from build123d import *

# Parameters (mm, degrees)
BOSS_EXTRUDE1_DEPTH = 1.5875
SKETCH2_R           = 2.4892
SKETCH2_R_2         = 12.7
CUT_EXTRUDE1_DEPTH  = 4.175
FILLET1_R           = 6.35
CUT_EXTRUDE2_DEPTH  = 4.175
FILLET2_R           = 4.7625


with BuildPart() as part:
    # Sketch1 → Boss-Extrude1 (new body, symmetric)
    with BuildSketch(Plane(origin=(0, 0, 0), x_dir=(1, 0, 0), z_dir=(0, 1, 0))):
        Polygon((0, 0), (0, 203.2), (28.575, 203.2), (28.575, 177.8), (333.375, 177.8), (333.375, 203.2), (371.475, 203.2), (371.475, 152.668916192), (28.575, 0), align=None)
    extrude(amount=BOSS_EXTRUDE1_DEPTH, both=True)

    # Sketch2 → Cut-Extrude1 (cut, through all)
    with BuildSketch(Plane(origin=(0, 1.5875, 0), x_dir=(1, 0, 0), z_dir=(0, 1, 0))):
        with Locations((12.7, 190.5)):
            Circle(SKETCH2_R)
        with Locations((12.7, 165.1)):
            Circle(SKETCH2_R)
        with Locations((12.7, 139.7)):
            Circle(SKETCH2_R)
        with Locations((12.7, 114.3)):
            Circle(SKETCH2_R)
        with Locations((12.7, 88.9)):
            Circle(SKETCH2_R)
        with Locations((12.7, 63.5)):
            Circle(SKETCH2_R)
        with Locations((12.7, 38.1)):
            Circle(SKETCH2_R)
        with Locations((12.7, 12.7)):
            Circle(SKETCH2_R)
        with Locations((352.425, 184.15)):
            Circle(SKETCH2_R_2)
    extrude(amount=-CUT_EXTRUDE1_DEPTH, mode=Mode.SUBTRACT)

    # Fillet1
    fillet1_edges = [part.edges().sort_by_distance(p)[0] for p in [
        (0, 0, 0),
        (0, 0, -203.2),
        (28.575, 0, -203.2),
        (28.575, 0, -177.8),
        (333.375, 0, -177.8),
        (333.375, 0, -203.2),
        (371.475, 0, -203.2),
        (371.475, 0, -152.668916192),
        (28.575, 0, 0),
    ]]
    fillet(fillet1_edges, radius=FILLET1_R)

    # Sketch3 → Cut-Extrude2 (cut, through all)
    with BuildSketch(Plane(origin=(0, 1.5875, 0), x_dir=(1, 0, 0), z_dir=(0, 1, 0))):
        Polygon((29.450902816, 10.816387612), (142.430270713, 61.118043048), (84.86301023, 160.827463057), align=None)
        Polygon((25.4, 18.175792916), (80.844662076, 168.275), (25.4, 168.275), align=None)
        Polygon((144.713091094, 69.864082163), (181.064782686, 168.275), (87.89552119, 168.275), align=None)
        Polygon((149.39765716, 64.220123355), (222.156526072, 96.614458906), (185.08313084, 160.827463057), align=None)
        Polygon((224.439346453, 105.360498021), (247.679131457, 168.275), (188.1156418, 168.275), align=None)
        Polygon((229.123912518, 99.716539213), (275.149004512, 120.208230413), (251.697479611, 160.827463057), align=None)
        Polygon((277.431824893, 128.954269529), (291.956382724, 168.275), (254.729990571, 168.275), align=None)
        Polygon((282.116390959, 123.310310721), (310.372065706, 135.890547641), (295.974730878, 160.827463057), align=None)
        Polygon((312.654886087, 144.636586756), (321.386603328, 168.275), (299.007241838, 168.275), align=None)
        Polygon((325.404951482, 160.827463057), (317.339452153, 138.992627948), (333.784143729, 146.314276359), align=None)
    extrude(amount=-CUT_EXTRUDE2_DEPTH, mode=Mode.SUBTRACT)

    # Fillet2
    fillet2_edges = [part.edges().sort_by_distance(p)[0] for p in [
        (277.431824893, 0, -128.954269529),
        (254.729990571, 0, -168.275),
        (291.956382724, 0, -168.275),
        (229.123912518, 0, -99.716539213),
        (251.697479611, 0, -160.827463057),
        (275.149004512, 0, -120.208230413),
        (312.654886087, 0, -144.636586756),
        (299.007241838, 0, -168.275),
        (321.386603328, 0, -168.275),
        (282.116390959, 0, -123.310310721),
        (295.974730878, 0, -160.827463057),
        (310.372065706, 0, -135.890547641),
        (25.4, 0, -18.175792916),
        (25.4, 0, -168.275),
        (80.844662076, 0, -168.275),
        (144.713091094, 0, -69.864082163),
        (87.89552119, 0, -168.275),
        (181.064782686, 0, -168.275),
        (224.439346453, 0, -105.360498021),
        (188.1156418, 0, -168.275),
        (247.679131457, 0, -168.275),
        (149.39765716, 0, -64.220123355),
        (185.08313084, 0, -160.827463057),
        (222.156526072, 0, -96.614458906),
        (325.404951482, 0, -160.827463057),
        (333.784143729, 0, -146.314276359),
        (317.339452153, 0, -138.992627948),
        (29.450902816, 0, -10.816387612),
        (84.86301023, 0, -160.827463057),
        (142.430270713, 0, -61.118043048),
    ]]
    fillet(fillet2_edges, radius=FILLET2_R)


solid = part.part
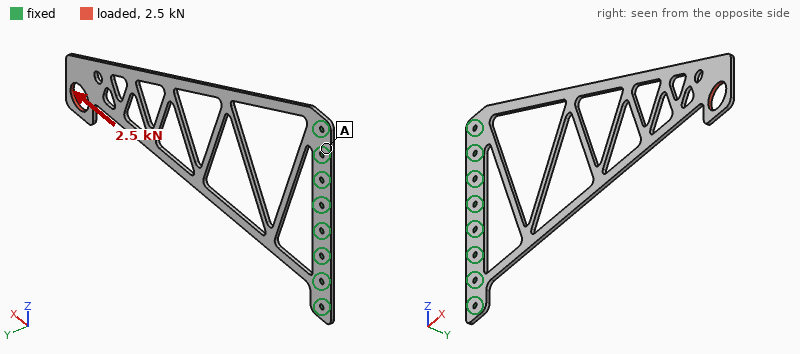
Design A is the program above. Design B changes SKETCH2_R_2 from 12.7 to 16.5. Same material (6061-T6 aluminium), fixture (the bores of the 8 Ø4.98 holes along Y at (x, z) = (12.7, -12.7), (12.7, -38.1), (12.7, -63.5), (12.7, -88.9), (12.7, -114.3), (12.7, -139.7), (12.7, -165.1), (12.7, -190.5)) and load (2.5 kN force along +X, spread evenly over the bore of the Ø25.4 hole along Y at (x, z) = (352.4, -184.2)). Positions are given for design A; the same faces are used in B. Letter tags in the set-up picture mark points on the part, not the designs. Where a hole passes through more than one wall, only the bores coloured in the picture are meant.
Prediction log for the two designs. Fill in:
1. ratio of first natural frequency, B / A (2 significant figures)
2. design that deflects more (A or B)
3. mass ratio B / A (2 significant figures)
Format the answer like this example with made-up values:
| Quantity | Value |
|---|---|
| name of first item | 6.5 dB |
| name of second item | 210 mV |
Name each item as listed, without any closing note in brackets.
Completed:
| Quantity | Value |
|---|---|
| ratio of first natural frequency, B / A | 1.0 |
| design that deflects more | B |
| mass ratio B / A | 0.98 |
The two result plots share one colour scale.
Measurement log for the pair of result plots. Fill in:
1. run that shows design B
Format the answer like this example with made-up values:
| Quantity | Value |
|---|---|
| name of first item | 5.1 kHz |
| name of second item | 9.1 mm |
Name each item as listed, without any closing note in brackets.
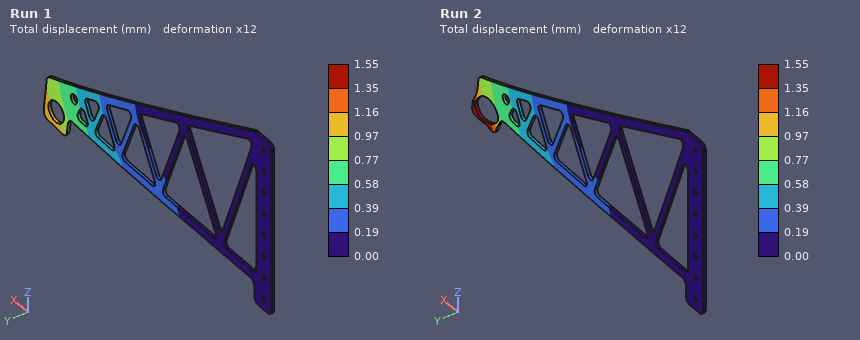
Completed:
| Quantity | Value |
|---|---|
| run that shows design B | Run 2 |
